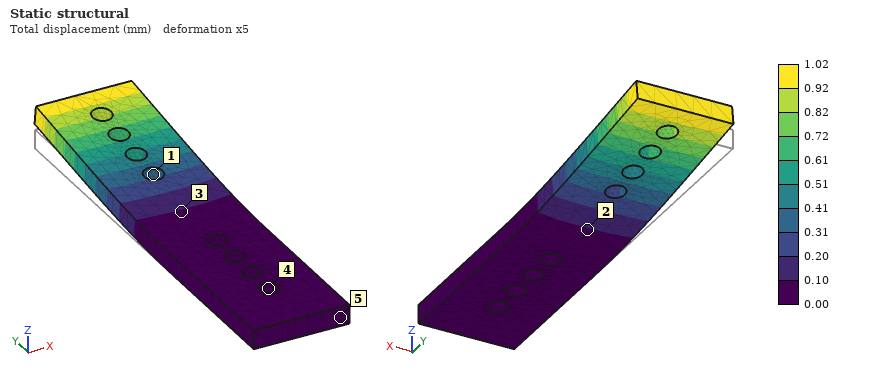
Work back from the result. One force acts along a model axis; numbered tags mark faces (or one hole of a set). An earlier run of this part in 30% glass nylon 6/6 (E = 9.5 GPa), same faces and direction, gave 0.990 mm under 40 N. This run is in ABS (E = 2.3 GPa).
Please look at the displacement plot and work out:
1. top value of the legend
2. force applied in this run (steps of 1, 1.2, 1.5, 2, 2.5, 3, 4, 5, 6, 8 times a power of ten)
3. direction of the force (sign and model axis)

1.02 mm
10 N
+Z
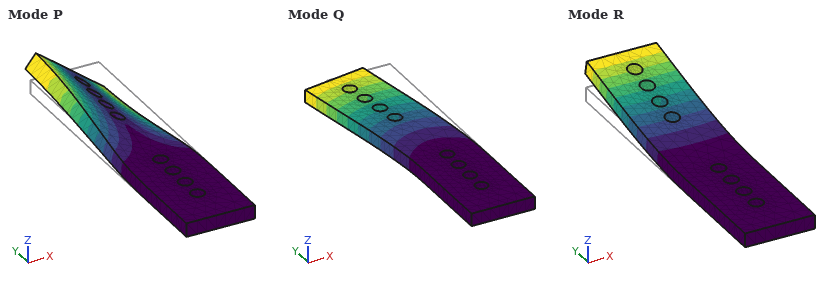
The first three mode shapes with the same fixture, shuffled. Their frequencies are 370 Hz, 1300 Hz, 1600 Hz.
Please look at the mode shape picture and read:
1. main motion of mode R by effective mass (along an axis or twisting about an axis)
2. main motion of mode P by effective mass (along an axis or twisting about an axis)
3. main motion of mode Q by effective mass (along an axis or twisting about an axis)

along Z
twisting about Y
along X
